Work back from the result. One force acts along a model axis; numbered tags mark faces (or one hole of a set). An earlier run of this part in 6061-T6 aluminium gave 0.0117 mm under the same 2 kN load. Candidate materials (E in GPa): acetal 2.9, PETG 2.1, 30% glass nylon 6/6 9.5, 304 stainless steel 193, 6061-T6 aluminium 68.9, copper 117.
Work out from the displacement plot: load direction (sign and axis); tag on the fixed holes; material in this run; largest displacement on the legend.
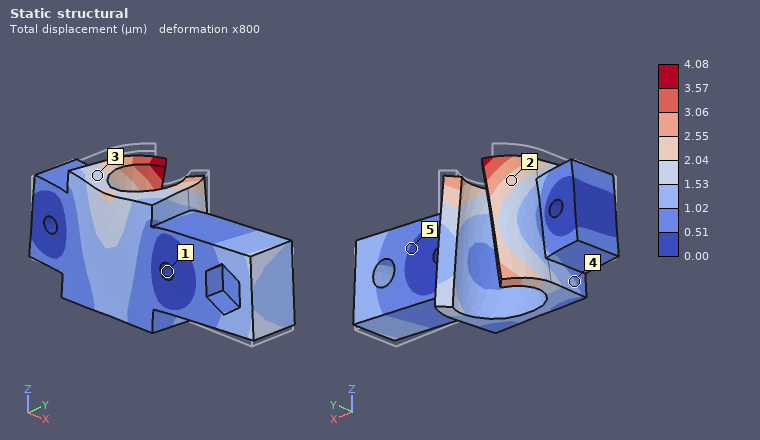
-Z
1
304 stainless steel
4.08 µm
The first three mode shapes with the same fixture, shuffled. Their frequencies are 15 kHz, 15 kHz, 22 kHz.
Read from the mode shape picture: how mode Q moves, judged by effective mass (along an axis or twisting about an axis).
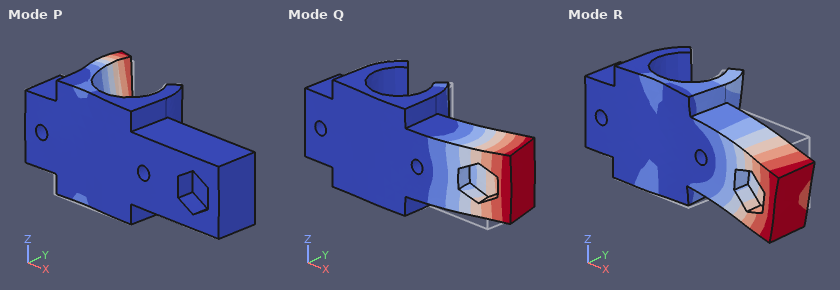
along Y
